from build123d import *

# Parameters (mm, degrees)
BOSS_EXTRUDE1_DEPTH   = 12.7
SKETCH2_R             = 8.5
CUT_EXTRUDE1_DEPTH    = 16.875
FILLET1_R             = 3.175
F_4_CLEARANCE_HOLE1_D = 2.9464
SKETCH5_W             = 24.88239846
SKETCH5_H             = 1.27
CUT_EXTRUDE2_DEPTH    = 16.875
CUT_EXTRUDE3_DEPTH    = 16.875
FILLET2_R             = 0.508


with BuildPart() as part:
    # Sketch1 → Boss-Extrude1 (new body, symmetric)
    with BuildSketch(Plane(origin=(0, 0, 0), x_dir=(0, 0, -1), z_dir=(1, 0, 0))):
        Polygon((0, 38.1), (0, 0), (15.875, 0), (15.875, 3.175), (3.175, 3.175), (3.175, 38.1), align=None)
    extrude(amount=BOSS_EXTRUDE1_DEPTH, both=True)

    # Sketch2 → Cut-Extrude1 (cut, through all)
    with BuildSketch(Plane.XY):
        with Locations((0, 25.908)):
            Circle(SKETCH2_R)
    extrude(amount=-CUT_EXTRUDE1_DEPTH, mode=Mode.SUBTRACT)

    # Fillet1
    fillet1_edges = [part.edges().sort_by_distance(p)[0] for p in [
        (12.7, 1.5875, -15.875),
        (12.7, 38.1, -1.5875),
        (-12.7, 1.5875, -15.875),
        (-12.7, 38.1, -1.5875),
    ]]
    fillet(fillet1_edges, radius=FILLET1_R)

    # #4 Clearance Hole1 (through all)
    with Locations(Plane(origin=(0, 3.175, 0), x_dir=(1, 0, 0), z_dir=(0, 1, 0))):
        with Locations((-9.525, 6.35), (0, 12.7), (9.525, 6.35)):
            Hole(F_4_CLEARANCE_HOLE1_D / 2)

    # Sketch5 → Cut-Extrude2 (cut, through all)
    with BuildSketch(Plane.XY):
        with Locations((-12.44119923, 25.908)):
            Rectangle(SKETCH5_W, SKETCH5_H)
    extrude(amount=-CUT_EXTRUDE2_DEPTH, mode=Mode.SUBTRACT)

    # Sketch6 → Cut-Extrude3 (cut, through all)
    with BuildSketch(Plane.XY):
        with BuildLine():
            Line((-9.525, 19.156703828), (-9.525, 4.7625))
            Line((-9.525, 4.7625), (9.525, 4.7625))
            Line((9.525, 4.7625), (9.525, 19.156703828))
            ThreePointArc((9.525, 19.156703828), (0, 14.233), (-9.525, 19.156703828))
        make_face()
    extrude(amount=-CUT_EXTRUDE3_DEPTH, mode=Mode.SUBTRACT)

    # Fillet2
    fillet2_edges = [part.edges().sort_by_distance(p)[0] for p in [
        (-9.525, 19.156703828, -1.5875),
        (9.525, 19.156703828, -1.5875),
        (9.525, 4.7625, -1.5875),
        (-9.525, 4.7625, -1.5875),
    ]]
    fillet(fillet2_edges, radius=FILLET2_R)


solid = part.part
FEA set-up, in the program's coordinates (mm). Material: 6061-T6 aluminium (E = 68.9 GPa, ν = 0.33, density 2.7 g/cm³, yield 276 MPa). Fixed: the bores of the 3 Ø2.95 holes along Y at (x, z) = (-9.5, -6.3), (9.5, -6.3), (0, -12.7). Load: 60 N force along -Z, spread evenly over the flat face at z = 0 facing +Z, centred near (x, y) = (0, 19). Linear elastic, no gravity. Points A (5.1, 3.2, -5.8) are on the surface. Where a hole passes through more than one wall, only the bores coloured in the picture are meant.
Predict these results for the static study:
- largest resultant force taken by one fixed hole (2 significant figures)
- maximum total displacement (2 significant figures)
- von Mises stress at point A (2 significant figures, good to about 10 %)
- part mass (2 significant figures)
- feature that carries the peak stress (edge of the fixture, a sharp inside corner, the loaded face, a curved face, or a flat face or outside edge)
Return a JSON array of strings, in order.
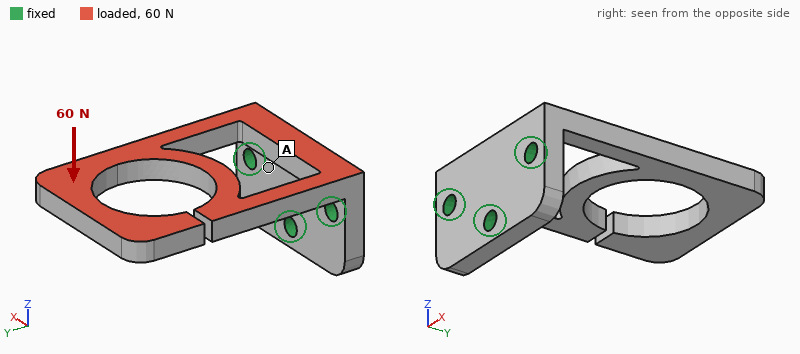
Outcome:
["29 N", "0.54 mm", "12 MPa", "7.0 g", "the loaded face"]
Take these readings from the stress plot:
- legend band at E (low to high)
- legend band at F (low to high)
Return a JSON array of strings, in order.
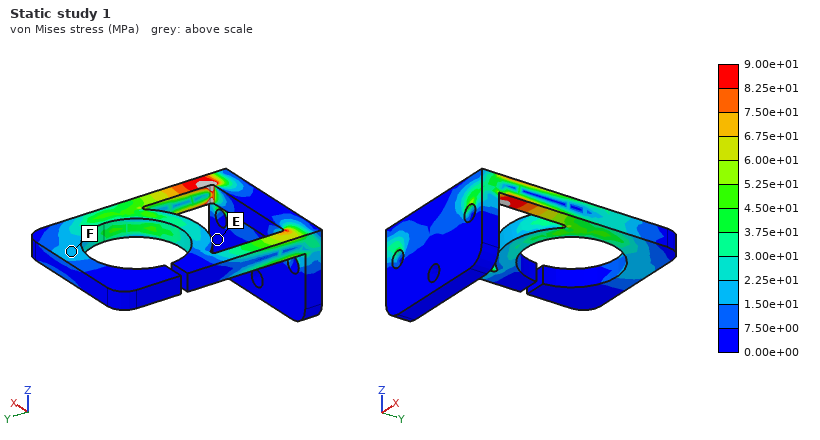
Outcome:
["0.00e+00 to 7.50e+00 MPa", "1.50e+01 to 2.25e+01 MPa"]
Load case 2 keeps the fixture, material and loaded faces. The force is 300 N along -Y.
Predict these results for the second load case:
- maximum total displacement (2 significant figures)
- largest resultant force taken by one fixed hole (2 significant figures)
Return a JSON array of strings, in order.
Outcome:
["0.53 mm", "170 N"]
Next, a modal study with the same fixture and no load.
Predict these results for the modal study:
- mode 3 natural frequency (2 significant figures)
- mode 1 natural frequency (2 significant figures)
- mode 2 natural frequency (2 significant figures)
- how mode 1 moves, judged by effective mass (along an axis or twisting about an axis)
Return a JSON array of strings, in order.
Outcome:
["2500 Hz", "970 Hz", "1800 Hz", "along Z"]
